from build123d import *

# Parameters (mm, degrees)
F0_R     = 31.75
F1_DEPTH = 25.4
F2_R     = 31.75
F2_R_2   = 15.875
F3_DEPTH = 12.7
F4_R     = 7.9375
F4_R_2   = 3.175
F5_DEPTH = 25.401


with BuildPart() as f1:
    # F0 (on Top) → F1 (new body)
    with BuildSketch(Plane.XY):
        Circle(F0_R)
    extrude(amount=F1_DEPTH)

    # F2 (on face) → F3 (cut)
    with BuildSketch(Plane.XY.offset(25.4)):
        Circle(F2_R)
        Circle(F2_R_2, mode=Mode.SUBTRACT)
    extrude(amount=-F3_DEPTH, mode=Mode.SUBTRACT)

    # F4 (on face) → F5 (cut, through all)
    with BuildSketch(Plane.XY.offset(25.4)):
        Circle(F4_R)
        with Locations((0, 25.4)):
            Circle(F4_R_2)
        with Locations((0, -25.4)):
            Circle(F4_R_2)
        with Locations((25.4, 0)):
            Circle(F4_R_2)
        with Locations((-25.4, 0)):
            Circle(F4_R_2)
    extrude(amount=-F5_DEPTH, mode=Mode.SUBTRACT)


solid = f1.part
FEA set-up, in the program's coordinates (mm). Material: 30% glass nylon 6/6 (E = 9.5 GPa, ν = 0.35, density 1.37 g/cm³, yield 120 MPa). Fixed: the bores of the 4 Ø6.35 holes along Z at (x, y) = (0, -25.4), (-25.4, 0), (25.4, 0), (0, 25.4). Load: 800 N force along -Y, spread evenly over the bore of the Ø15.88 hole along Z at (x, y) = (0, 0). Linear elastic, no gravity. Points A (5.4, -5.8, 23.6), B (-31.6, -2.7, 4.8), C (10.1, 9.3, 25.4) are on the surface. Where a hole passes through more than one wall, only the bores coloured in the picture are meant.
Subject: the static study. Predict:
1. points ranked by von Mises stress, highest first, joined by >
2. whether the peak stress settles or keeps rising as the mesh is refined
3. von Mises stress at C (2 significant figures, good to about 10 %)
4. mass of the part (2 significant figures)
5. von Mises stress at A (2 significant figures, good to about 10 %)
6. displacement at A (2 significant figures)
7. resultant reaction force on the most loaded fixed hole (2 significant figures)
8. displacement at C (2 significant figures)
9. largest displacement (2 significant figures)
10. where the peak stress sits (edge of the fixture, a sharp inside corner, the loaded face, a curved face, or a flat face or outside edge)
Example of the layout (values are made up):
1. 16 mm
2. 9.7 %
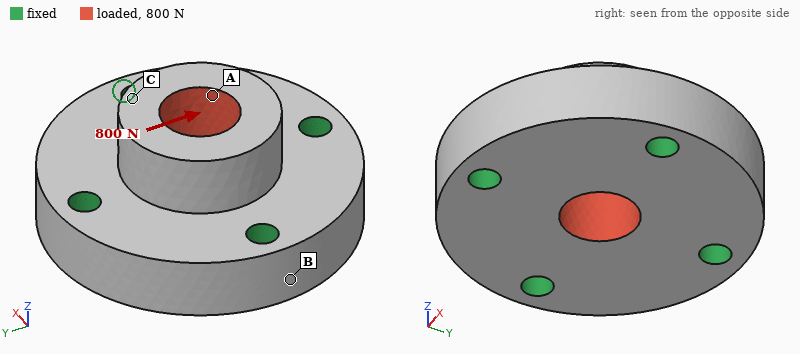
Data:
1. A > C > B
2. keeps rising
3. 0.71 MPa
4. 60 g
5. 1.2 MPa
6. 5.7 µm
7. 280 N
8. 5.5 µm
9. 6.5 µm
10. edge of the fixture
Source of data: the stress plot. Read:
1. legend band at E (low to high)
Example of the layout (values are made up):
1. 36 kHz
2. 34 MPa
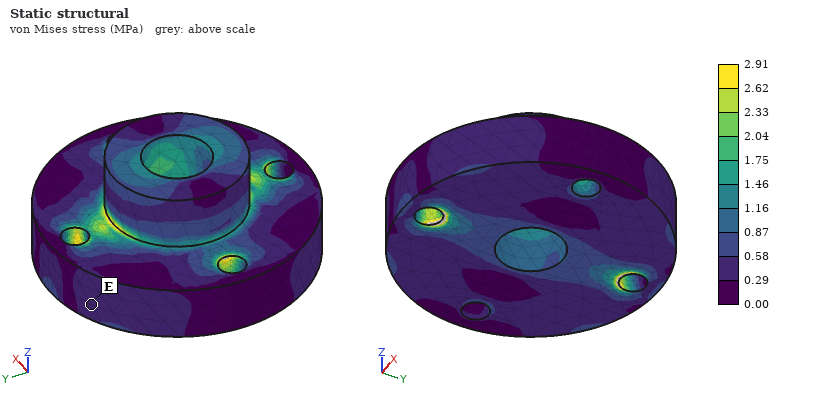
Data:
1. 0.29 to 0.58 MPa
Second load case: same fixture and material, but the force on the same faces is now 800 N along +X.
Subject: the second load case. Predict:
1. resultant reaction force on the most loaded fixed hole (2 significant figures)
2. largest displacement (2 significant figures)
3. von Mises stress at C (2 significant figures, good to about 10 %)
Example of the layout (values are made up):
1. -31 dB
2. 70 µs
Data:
1. 280 N
2. 6.5 µm
3. 0.75 MPa
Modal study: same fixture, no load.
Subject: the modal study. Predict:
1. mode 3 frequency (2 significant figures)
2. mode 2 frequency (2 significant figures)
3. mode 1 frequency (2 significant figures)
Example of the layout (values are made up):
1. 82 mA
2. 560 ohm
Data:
1. 13 kHz
2. 13 kHz
3. 13 kHz
